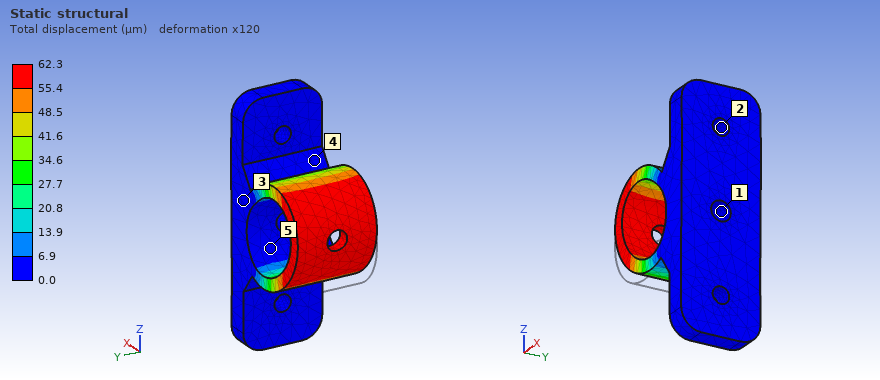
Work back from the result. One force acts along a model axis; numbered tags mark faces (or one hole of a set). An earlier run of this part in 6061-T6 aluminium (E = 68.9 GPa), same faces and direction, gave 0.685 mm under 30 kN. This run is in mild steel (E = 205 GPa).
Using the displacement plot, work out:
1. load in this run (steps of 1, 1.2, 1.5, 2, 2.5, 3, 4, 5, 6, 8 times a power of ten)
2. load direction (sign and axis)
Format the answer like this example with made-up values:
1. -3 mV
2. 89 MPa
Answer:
1. 8 kN
2. +Z
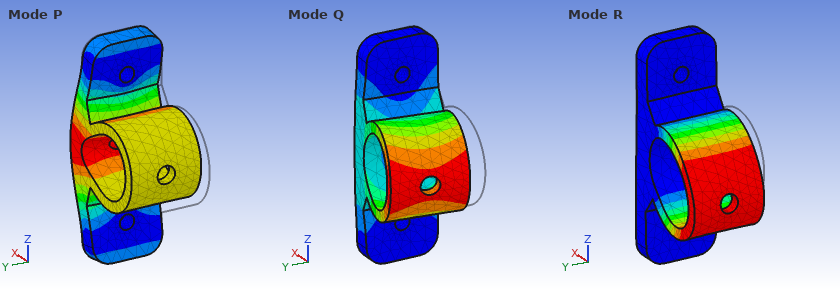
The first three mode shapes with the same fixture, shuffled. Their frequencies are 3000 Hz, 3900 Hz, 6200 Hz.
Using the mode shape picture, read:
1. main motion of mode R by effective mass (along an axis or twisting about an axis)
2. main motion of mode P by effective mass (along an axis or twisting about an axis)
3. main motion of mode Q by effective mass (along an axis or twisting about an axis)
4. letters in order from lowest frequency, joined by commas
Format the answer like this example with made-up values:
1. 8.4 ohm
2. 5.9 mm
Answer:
1. along Z
2. along X
3. along Y
4. Q, R, P
